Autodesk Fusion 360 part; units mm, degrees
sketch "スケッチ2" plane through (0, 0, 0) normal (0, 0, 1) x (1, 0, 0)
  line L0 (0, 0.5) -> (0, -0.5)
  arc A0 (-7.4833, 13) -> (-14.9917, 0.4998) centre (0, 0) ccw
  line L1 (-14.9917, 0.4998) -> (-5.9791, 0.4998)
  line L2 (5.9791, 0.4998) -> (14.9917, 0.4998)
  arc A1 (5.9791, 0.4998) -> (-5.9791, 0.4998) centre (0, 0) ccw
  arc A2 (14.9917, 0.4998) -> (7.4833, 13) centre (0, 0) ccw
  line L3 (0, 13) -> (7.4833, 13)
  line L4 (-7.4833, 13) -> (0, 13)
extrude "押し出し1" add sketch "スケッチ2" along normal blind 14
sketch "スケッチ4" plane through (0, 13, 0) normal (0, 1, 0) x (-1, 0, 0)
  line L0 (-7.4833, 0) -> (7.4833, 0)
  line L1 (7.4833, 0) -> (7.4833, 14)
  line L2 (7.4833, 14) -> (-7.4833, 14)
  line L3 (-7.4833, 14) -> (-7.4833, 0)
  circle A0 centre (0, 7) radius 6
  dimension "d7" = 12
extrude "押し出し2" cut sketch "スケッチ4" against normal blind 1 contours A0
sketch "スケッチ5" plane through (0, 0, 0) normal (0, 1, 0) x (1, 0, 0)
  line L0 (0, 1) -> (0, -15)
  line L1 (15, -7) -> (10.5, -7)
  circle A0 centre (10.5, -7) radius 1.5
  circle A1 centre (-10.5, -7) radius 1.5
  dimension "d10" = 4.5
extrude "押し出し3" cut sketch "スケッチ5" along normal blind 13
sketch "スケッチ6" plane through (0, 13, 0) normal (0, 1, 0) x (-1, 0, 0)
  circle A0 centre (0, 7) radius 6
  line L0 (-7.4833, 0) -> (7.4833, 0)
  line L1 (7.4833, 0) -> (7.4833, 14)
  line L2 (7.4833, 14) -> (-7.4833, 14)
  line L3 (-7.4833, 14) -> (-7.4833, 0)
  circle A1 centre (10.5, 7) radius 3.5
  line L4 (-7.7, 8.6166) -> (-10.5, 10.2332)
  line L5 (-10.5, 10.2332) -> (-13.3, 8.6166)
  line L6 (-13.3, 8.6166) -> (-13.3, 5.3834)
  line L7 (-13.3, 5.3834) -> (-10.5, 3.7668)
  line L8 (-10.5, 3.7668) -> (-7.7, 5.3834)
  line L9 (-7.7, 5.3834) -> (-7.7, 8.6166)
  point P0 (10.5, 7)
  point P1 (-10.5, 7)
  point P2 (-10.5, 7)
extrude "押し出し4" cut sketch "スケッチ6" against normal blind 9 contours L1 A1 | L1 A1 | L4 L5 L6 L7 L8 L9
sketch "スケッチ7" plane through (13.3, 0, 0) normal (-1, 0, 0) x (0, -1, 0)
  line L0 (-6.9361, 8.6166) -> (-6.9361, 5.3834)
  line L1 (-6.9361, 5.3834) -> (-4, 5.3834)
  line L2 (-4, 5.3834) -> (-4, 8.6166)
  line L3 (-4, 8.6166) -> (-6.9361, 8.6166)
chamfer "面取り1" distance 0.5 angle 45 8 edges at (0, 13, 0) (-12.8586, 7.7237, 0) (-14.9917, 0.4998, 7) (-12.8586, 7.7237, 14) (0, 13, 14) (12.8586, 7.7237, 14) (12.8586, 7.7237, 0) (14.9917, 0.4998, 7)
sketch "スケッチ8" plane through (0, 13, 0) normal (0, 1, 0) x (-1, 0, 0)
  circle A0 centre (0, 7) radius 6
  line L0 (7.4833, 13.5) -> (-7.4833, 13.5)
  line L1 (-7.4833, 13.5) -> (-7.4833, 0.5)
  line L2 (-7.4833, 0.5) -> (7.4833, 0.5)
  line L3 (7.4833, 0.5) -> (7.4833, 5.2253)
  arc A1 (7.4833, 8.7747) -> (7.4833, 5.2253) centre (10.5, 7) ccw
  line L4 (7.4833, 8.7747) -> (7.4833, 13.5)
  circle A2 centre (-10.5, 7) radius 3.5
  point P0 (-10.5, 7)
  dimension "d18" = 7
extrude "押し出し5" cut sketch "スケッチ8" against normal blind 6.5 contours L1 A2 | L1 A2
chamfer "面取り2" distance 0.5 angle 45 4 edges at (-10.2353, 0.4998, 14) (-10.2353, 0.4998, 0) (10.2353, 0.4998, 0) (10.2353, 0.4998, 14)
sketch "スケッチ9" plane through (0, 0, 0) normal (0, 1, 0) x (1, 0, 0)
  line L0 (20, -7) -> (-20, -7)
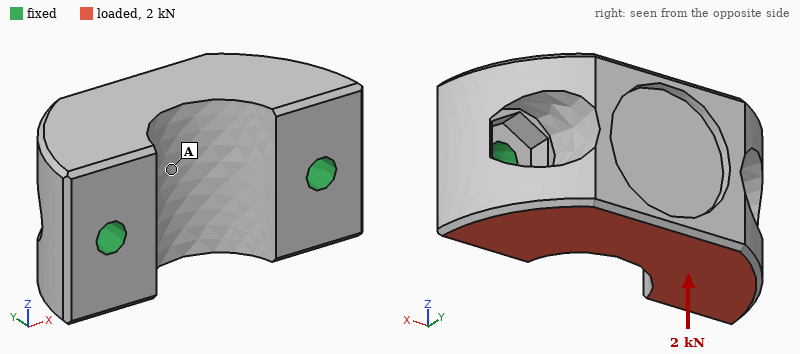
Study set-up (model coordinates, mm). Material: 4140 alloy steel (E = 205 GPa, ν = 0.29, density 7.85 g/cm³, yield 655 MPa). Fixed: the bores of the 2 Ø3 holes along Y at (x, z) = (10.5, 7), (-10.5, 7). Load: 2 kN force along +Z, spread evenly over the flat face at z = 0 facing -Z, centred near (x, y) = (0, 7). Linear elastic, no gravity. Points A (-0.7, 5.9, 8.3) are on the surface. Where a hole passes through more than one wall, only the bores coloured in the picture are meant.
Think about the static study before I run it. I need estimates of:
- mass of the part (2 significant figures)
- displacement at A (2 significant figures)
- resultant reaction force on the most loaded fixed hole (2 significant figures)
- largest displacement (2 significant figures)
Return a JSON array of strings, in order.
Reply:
["24 g", "4.9 µm", "1.0 kN", "13 µm"]
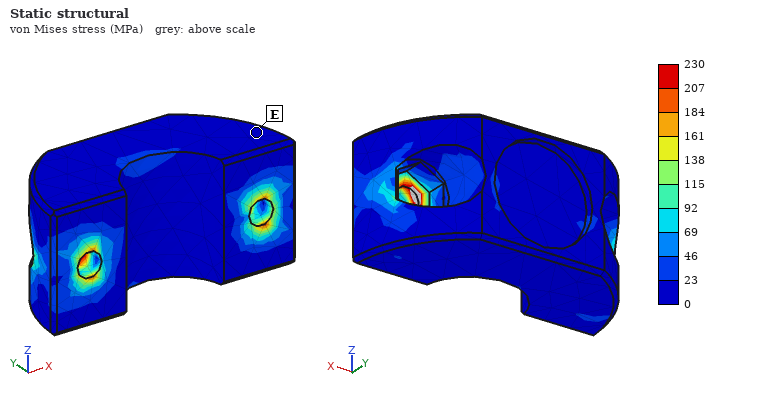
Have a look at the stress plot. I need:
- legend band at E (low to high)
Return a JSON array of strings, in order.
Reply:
["0 to 23 MPa"]
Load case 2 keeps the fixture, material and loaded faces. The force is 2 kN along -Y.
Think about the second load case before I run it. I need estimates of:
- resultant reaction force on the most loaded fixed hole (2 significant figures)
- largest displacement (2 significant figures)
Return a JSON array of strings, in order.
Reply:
["1.1 kN", "17 µm"]
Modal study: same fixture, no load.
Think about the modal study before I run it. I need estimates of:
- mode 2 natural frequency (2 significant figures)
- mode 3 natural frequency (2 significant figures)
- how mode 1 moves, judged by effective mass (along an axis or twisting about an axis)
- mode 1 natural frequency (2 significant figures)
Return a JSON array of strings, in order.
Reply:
["38 kHz", "38 kHz", "along Z", "15 kHz"]
